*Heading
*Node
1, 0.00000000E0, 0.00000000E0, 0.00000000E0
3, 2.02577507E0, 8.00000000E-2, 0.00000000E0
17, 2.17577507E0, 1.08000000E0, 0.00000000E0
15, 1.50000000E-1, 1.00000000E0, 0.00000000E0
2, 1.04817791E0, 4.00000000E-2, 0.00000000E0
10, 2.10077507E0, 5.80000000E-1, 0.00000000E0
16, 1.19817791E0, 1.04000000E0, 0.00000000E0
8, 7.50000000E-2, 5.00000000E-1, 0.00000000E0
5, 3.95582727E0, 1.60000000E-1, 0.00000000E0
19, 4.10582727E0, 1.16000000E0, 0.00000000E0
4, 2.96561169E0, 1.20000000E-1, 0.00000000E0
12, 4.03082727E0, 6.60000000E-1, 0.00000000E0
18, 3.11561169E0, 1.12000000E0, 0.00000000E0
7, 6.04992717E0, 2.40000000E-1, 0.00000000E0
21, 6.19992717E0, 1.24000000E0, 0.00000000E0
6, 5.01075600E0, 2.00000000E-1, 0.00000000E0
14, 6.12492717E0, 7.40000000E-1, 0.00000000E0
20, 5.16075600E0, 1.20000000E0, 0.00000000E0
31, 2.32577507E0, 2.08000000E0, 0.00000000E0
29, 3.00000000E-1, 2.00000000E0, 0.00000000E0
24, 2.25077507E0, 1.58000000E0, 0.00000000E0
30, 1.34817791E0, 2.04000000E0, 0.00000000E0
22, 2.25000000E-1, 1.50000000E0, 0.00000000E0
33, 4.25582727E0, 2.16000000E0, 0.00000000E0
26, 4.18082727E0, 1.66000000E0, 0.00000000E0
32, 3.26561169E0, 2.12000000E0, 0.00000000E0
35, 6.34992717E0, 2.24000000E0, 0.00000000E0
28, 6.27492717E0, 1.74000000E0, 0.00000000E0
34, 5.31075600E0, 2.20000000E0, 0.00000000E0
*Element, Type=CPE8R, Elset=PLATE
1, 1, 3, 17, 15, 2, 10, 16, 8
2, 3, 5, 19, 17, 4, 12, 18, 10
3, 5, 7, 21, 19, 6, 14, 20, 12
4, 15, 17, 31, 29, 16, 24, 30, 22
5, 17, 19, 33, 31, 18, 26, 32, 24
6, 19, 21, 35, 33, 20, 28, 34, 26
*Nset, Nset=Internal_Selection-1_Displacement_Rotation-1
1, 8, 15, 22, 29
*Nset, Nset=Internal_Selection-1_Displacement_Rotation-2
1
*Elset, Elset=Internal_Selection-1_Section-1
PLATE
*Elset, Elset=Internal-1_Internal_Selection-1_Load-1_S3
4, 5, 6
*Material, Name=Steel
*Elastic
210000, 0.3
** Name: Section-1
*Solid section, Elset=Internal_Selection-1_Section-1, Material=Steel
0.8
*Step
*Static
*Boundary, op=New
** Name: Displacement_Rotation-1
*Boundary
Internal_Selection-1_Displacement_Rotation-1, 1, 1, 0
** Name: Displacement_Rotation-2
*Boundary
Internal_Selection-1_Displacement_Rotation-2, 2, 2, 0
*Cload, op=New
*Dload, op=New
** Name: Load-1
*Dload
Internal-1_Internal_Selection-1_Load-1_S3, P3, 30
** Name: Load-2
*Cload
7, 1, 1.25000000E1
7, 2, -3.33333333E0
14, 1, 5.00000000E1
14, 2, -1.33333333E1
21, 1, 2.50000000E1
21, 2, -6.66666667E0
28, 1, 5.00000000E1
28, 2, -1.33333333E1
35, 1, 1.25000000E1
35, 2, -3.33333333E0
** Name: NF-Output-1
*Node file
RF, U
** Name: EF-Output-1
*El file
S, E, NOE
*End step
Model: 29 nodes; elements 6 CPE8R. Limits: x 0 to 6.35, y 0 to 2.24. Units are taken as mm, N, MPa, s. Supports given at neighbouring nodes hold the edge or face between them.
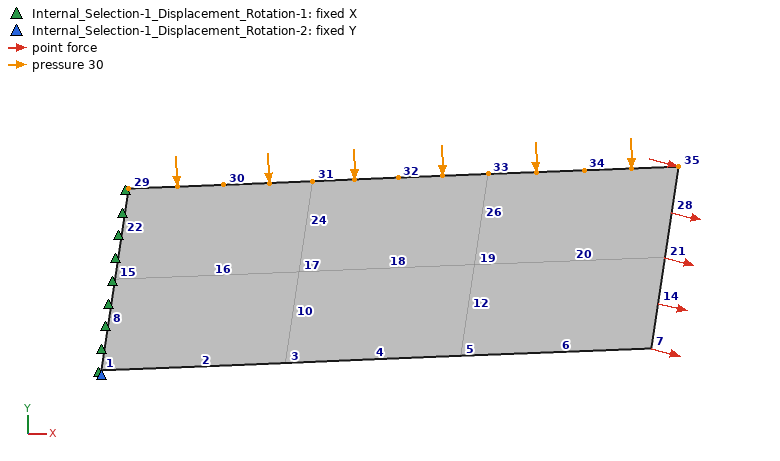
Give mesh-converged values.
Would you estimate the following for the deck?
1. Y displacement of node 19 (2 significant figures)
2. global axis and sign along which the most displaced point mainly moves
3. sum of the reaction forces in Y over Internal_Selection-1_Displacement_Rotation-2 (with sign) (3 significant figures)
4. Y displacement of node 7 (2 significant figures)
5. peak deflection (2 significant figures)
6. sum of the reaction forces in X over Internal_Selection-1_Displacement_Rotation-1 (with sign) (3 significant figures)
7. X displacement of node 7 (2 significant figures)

-0.041 mm
-Y
185 N
-0.071 mm
0.079 mm
-156 N
-0.0098 mm
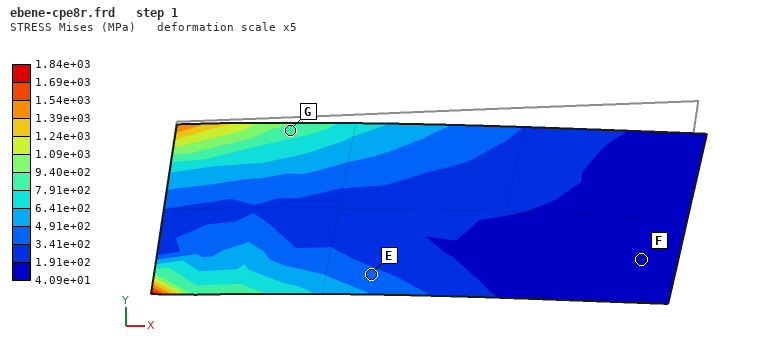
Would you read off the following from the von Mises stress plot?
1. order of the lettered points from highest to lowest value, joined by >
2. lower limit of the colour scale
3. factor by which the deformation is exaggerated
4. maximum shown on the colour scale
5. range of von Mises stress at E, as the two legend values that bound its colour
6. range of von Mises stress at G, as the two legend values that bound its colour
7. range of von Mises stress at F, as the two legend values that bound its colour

G > E > F
4.09e+01 MPa
5
1.84e+03 MPa
3.41e+02 to 4.91e+02 MPa
7.91e+02 to 9.40e+02 MPa
4.09e+01 to 1.91e+02 MPa
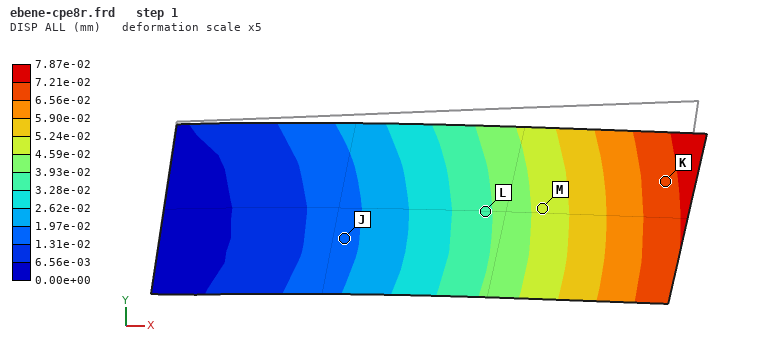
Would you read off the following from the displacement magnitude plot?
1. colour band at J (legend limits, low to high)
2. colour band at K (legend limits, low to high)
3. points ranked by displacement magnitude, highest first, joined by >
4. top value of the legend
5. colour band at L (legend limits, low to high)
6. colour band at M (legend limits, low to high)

1.31e-02 to 1.97e-02 mm
6.56e-02 to 7.21e-02 mm
K > M > L > J
7.87e-02 mm
3.28e-02 to 3.93e-02 mm
4.59e-02 to 5.24e-02 mm
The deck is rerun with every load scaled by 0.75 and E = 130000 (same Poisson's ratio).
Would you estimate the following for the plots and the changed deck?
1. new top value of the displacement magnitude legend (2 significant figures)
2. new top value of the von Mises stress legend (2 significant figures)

0.095 mm
1400 MPa
